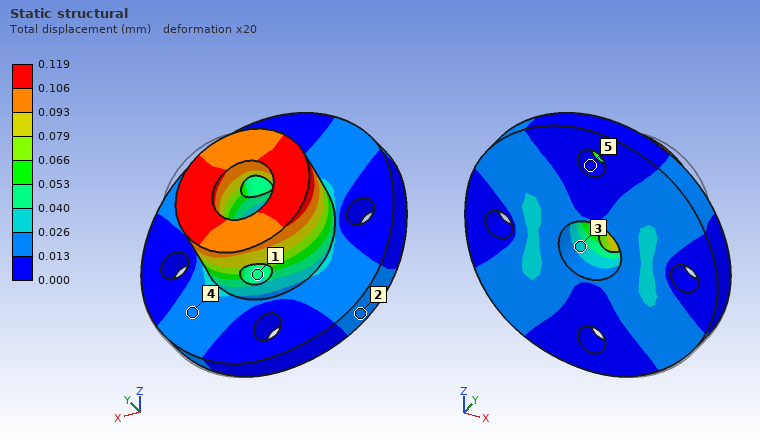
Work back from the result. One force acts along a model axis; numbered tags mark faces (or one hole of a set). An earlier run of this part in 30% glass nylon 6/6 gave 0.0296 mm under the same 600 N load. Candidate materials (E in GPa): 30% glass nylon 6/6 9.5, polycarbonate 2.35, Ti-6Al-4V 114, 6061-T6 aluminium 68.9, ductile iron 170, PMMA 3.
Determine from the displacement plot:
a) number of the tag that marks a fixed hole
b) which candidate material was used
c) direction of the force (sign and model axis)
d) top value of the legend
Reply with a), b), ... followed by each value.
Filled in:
a) 5
b) polycarbonate
c) -X
d) 0.119 mm
